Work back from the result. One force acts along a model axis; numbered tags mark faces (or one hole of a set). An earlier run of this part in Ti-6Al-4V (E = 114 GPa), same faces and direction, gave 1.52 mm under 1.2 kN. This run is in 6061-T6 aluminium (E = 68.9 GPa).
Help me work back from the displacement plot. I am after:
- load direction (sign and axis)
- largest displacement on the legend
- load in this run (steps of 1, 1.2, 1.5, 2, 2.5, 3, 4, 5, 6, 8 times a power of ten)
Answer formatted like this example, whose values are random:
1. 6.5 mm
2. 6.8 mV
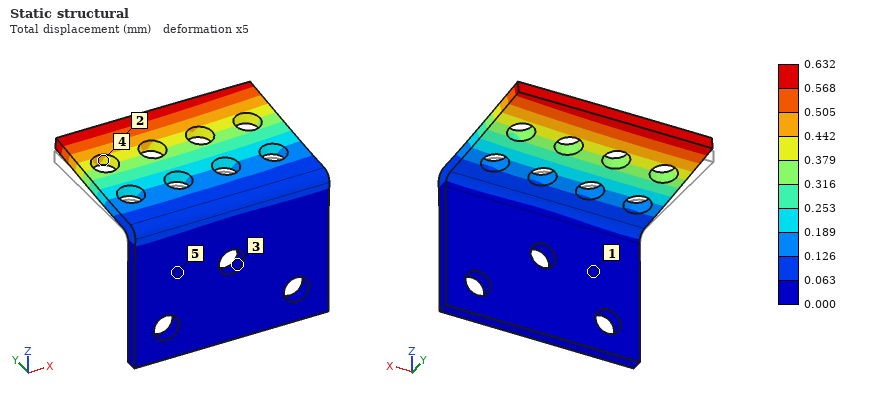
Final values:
1. +Z
2. 0.632 mm
3. 300 N
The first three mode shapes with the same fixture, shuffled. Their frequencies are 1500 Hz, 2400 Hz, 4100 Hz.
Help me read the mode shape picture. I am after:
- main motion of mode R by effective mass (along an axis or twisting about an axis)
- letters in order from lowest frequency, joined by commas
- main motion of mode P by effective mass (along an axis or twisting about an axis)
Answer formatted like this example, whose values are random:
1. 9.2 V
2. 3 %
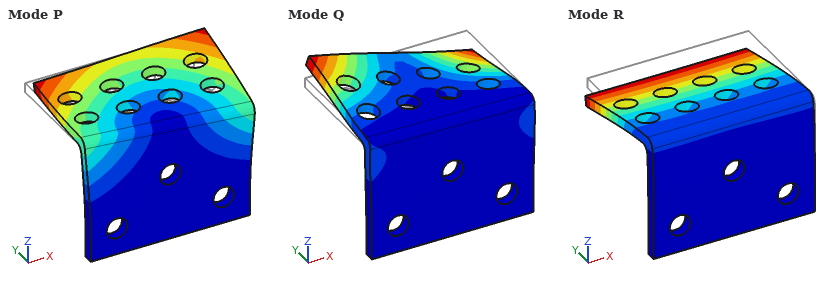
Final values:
1. along Z
2. R, P, Q
3. along X
